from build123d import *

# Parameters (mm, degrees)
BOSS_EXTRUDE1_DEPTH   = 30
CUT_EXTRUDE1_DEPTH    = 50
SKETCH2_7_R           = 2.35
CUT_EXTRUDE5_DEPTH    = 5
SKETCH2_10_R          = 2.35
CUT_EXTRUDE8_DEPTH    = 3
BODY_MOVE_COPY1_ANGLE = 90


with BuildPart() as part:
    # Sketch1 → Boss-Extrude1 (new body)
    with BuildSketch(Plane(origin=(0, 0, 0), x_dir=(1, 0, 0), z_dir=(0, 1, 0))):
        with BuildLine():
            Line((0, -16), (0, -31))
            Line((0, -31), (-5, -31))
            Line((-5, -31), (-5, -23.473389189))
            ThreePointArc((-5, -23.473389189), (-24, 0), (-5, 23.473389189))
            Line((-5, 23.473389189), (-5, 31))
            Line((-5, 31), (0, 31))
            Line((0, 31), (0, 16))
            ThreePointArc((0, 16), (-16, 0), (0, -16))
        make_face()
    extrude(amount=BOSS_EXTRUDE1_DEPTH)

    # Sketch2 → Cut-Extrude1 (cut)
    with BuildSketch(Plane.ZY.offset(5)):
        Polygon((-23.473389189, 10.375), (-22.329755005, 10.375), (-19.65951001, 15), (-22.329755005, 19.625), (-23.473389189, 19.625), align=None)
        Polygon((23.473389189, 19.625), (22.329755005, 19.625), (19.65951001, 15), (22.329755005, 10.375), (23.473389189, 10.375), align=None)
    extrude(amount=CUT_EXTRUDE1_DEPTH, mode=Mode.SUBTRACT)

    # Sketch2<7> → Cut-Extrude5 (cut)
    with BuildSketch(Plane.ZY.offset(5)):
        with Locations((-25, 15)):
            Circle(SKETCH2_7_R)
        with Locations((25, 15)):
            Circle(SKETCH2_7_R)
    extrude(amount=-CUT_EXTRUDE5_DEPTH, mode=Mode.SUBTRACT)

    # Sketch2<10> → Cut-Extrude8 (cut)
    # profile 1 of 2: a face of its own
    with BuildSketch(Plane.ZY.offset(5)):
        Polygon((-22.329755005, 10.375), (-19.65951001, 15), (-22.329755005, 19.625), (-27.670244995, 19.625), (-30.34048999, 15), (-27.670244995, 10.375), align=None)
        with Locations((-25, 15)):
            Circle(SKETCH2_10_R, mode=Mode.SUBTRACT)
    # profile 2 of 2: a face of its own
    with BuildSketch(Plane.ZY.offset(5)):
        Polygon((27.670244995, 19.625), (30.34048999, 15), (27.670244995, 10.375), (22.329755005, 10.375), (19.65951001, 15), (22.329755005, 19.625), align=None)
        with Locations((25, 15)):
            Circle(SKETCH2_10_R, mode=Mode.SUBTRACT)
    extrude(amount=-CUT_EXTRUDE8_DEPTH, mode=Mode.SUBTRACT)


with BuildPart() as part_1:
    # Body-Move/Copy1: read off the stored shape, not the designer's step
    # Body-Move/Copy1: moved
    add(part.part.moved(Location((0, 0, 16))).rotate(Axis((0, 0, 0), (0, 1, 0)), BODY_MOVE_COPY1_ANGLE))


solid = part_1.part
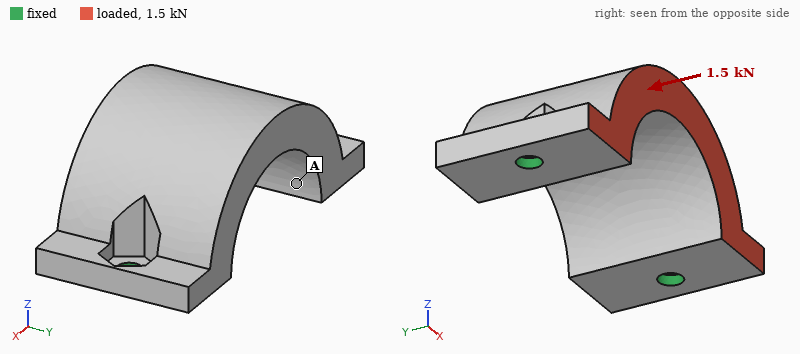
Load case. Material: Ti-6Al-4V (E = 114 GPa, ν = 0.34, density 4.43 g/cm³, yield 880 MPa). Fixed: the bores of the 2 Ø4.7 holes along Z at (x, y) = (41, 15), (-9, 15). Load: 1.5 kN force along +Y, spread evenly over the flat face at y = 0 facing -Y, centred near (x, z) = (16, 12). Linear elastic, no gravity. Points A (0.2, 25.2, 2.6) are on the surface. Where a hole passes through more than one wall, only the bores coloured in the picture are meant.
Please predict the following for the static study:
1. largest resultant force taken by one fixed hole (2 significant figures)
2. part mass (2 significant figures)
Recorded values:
750 N
73 g
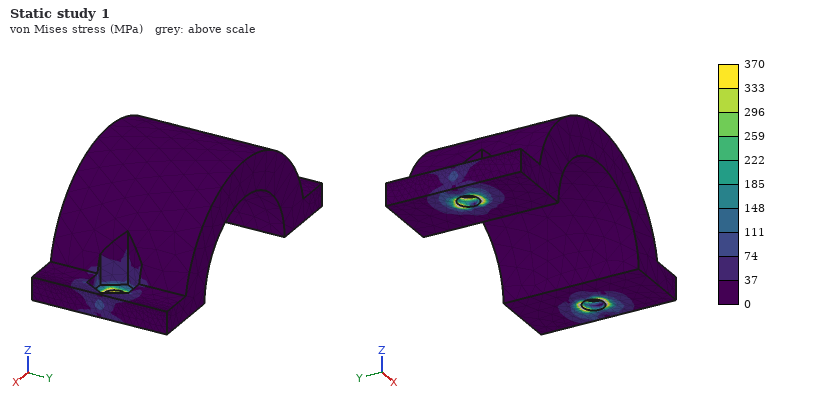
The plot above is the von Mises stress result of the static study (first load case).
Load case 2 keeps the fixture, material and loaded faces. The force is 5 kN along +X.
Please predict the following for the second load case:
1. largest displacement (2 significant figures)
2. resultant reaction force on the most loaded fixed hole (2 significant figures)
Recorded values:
47 µm
3.0 kN
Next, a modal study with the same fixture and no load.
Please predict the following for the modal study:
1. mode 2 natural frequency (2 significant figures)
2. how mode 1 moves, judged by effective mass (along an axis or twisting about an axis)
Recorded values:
11 kHz
along Y
